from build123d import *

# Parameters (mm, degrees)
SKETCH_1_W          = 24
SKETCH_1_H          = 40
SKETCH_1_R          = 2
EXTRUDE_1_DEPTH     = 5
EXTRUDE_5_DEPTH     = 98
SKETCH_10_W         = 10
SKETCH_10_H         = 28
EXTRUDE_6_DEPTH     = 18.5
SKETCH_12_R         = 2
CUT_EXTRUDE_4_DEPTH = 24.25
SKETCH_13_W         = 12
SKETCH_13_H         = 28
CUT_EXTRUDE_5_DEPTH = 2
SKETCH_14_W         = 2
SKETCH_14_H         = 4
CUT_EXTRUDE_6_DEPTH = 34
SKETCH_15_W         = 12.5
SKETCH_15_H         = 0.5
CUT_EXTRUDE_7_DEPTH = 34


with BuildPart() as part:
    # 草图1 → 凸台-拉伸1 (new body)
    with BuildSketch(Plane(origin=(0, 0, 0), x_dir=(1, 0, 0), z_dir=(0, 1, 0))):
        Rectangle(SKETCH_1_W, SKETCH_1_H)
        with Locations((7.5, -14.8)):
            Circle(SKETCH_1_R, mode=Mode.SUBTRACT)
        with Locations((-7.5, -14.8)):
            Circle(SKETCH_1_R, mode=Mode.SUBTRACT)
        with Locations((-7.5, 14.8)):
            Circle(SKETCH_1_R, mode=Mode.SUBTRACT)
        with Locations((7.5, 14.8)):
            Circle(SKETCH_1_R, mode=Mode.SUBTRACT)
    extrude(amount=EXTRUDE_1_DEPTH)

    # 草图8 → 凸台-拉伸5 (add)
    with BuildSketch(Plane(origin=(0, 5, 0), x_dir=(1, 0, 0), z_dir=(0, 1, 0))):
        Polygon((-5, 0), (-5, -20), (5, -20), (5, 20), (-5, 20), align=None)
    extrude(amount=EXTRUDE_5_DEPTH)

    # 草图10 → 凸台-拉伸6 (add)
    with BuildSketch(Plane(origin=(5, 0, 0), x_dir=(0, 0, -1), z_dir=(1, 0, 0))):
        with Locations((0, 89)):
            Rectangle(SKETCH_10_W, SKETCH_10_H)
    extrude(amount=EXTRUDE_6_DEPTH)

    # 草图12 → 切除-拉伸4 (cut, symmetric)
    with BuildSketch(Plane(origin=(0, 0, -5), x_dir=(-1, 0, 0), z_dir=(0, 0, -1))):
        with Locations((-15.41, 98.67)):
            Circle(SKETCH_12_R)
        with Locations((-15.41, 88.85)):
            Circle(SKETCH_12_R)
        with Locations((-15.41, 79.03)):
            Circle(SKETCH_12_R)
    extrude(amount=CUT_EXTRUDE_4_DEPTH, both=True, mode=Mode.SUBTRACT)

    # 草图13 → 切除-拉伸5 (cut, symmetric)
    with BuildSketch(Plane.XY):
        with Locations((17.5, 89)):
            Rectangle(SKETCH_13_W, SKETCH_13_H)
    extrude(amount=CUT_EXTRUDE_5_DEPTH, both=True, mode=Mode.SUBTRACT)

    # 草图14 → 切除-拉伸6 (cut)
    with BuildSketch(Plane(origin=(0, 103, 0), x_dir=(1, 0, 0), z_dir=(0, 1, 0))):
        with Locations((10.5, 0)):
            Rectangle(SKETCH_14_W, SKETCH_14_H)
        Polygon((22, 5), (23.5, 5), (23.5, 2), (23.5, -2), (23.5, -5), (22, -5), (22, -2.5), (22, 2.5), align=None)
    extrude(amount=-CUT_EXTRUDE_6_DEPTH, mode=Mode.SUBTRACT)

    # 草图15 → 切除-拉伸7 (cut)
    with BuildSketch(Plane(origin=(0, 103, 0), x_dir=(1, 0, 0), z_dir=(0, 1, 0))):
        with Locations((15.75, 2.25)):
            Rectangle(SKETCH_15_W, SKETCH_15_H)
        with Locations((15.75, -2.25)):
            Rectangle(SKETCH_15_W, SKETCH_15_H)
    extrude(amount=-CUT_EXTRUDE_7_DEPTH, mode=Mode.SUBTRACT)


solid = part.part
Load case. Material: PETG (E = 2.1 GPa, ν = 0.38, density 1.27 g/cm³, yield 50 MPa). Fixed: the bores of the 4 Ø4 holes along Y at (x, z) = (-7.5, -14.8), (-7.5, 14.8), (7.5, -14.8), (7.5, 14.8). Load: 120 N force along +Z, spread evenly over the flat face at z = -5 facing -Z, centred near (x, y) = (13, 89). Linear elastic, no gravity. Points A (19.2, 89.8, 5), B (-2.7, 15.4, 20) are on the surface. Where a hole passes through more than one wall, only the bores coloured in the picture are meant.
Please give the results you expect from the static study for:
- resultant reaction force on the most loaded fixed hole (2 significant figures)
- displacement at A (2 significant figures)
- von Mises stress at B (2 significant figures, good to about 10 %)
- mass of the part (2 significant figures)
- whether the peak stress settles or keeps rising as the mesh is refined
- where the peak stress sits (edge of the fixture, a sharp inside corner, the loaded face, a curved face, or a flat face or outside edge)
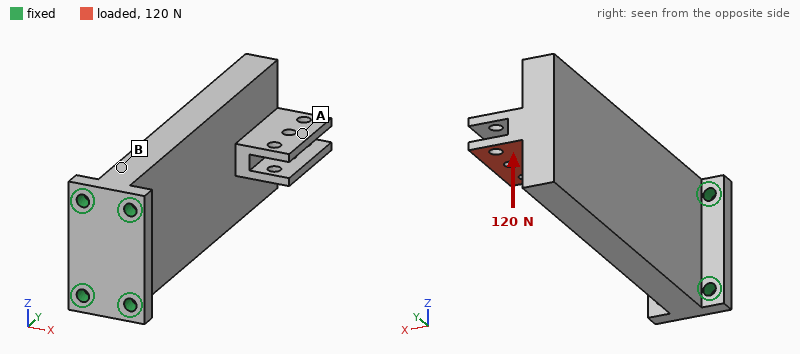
220 N
0.62 mm
4.1 MPa
59 g
keeps rising
edge of the fixture
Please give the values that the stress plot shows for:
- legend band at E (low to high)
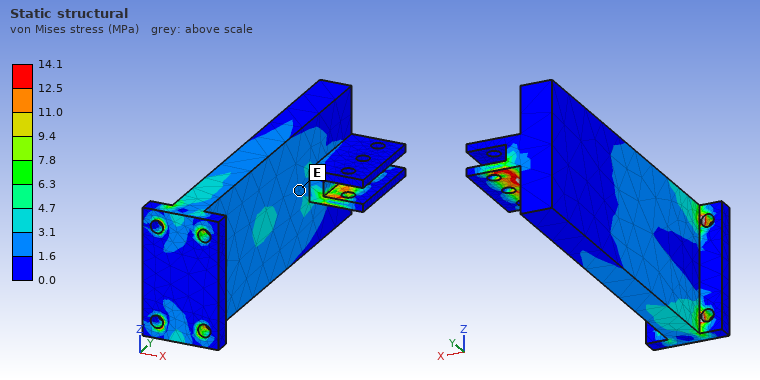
1.6 to 3.1 MPa
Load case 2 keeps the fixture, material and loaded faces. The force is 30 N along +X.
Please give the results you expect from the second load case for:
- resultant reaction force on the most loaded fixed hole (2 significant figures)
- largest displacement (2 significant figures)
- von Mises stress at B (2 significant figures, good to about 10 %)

100 N
1.3 mm
1.8 MPa
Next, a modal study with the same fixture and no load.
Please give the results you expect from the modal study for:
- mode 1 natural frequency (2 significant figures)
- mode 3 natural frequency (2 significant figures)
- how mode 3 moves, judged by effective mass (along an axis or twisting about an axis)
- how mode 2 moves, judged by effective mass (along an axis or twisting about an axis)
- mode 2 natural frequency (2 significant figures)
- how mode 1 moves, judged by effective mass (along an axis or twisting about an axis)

180 Hz
880 Hz
twisting about Y
along Z
590 Hz
along X
